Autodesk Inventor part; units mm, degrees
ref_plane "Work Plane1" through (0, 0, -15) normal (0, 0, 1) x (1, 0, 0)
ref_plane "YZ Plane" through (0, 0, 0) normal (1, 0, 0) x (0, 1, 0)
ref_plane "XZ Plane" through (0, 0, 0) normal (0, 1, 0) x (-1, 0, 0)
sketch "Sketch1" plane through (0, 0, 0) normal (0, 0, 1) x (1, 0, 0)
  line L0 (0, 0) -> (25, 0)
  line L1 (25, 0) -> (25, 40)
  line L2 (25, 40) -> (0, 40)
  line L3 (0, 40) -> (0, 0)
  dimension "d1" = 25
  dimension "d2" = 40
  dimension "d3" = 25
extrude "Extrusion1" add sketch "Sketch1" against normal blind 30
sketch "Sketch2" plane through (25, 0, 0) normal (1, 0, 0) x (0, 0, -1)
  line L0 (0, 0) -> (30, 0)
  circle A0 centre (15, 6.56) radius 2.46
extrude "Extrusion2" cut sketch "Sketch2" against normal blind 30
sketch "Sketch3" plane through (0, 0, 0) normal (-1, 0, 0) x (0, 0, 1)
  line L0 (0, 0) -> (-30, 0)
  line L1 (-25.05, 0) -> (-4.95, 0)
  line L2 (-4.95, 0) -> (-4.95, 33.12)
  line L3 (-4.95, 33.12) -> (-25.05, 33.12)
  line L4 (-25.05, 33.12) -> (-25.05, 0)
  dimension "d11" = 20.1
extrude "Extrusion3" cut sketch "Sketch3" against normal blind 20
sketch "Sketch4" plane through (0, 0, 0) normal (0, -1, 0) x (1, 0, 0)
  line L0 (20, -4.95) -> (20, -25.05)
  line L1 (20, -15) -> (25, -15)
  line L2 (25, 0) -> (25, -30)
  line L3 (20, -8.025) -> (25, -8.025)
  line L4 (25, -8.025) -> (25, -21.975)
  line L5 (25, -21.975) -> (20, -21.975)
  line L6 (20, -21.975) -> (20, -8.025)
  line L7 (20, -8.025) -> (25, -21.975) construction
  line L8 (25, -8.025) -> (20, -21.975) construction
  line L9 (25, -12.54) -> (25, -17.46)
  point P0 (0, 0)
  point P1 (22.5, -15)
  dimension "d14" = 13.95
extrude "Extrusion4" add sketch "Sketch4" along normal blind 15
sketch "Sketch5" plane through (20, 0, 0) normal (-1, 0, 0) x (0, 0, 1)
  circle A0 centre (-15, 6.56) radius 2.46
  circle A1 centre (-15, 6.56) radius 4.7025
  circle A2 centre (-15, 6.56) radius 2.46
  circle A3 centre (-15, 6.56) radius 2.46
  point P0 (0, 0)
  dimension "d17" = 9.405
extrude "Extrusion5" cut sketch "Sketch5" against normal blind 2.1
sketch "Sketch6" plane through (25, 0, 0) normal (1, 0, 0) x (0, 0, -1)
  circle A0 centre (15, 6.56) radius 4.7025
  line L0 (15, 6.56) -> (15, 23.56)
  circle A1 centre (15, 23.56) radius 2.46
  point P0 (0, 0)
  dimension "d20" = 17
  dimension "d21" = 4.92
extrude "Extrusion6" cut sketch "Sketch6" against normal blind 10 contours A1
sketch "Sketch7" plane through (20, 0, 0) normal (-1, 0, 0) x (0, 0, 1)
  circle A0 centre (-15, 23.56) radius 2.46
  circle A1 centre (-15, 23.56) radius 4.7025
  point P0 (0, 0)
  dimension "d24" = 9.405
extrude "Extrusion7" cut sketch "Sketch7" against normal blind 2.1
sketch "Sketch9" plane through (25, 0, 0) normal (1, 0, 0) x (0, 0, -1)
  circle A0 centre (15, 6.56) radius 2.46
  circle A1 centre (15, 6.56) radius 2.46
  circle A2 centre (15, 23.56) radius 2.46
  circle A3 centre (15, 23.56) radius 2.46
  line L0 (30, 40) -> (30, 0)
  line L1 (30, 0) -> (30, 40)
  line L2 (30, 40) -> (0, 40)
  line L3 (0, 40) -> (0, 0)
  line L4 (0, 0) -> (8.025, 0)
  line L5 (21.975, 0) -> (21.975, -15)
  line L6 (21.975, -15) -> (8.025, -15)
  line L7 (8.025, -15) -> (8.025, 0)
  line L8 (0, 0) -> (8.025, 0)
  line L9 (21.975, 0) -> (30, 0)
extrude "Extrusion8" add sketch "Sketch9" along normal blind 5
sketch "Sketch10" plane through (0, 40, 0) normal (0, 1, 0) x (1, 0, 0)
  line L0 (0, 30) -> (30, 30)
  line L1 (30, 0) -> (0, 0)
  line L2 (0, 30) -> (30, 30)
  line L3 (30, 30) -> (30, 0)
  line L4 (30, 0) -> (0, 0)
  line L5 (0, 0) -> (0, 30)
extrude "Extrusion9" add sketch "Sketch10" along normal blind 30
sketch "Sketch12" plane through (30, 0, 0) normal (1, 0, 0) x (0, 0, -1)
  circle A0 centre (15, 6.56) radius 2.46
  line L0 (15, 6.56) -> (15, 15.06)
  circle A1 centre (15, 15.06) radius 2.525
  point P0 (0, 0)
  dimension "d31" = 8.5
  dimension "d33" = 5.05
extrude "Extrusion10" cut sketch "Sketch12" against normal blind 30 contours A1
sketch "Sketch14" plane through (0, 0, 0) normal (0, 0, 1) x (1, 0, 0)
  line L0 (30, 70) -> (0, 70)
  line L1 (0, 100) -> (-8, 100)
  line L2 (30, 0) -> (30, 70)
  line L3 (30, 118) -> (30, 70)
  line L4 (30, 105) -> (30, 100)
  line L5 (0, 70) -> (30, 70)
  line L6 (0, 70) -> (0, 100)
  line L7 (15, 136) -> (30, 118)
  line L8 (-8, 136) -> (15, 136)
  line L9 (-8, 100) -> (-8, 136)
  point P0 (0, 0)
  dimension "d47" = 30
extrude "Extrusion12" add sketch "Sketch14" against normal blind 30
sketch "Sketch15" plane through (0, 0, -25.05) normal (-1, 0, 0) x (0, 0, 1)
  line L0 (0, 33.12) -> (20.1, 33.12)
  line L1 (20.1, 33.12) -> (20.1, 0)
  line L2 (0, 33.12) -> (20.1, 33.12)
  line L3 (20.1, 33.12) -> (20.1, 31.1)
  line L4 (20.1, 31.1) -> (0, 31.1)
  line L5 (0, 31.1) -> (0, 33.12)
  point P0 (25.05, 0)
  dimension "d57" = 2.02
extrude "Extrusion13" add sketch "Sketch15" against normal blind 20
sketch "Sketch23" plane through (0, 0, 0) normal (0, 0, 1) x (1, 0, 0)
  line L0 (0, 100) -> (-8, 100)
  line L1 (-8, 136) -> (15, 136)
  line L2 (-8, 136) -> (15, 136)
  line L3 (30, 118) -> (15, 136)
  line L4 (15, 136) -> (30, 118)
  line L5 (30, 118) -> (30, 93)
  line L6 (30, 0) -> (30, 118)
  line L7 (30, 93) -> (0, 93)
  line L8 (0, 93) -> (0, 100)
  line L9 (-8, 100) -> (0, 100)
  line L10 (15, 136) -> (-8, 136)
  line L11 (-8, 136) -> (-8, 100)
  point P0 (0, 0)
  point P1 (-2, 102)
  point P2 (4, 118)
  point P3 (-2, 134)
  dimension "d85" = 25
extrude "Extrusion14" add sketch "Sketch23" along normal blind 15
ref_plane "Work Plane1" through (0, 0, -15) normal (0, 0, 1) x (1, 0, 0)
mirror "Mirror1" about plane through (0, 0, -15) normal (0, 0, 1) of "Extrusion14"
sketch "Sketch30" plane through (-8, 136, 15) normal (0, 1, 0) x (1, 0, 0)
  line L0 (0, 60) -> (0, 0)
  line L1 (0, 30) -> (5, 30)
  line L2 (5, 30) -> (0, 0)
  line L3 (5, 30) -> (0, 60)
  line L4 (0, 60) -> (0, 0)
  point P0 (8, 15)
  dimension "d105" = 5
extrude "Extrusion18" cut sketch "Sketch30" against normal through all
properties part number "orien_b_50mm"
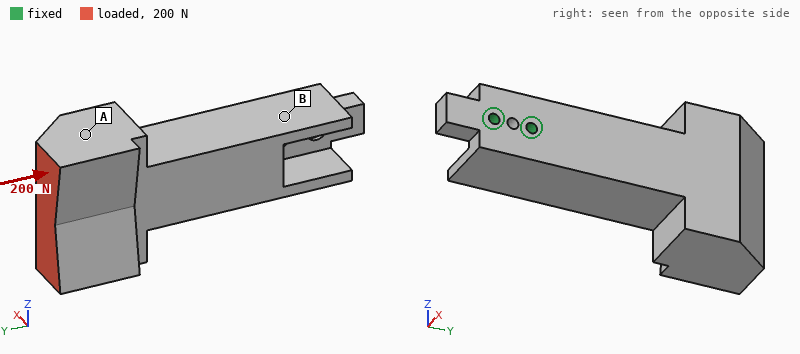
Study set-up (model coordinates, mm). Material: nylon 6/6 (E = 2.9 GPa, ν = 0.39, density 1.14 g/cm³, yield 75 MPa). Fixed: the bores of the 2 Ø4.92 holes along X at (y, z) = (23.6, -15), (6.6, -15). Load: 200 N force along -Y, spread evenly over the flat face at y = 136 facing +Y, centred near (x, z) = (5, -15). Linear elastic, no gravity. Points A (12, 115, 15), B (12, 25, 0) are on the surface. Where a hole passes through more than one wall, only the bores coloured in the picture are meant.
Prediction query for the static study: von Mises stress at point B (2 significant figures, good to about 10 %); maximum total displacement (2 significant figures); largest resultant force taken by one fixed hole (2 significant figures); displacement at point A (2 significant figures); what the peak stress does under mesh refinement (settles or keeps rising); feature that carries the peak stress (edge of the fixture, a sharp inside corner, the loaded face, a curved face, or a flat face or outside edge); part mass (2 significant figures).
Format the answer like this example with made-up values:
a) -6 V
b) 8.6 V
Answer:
a) 1.2 MPa
b) 0.31 mm
c) 200 N
d) 0.24 mm
e) keeps rising
f) edge of the fixture
g) 180 g
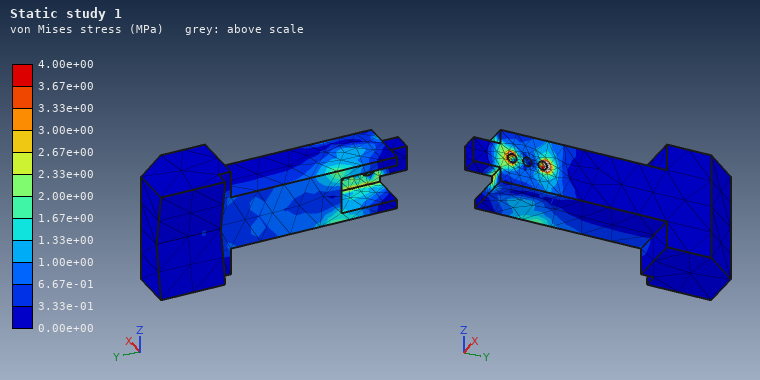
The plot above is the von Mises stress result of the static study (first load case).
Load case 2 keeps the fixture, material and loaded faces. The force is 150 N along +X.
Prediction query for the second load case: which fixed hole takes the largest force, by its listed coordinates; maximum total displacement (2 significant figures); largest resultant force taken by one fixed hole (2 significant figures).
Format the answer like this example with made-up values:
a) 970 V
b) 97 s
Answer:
a) (23.6, -15)
b) 1.4 mm
c) 820 N
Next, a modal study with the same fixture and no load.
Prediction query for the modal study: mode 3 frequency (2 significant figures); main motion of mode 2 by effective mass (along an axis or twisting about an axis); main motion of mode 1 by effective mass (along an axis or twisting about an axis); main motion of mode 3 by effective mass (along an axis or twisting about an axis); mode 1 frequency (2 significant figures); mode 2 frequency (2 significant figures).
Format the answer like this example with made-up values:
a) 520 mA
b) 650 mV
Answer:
a) 570 Hz
b) along Z
c) along X
d) twisting about Y
e) 210 Hz
f) 240 Hz
